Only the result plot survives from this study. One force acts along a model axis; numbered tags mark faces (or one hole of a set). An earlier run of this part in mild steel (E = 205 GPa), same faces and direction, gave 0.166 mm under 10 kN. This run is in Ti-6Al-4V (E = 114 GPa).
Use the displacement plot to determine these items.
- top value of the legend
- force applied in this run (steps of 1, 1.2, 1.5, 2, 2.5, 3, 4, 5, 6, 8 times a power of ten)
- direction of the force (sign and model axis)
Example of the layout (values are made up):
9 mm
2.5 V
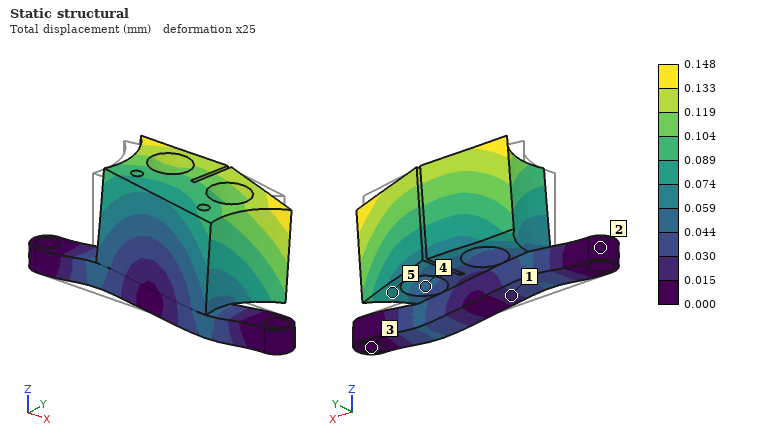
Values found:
0.148 mm
5 kN
+X
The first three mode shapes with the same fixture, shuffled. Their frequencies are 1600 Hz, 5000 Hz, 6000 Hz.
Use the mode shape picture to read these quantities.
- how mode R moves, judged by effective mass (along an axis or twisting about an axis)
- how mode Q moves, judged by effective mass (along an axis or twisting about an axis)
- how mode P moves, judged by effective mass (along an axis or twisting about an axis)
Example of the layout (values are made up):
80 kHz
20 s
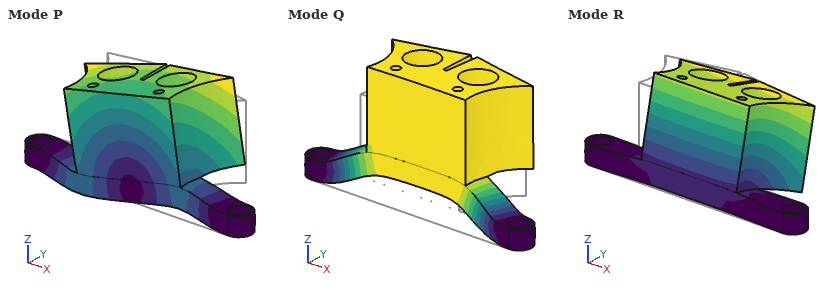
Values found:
along Y
along Z
along X
